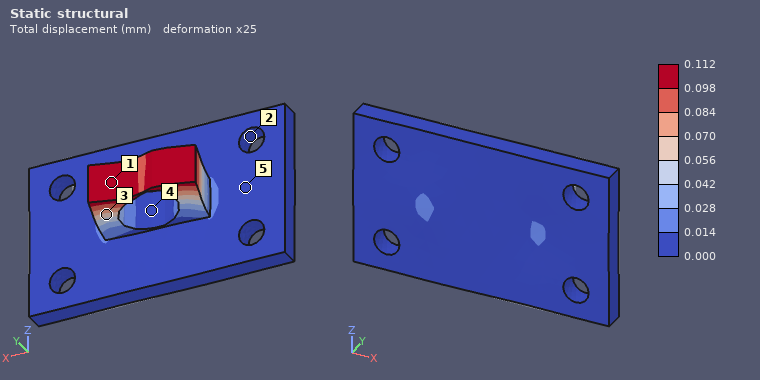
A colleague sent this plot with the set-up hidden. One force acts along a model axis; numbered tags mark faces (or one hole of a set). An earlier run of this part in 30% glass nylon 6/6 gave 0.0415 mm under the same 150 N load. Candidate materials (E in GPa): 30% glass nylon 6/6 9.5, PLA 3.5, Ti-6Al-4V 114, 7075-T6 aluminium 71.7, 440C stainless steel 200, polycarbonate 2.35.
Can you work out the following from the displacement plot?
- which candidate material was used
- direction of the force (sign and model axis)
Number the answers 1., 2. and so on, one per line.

1. PLA
2. -X
